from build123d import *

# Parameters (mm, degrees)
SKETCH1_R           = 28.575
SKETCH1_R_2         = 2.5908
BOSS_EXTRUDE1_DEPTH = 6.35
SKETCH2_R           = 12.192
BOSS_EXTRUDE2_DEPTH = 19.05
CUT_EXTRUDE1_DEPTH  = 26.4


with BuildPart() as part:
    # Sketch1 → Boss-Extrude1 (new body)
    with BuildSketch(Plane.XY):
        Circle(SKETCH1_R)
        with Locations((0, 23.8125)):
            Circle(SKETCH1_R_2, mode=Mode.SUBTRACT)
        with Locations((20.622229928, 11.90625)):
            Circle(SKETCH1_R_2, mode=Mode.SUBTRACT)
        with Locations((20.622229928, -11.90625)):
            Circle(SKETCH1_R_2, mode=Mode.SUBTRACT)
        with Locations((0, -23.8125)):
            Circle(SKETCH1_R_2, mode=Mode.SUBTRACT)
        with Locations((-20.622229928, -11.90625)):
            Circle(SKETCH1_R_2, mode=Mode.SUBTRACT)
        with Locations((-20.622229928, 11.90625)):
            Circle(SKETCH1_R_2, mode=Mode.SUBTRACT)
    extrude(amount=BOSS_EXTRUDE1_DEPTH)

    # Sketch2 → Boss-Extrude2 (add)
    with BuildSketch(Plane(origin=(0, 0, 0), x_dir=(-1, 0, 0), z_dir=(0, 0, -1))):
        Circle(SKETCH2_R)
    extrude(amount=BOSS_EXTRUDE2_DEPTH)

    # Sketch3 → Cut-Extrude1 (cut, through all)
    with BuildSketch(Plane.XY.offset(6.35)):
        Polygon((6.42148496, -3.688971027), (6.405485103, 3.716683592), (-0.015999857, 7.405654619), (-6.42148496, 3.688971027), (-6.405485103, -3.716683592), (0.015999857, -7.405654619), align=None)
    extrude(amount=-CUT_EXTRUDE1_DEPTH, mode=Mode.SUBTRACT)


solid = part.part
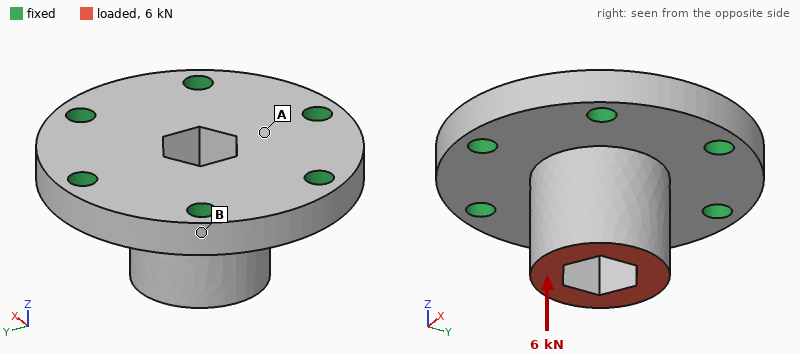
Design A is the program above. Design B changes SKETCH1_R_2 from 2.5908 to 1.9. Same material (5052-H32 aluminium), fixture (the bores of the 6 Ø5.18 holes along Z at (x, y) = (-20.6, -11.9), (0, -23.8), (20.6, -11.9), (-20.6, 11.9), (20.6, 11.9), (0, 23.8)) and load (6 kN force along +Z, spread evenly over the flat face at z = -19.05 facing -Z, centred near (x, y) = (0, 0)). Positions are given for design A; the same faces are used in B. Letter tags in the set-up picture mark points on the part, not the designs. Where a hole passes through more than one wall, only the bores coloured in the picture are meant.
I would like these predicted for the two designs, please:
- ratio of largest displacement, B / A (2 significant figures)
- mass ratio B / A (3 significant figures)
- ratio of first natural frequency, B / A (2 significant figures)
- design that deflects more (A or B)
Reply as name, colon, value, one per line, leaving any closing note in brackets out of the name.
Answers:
ratio of largest displacement, B / A: 1.1
mass ratio B / A: 1.02
ratio of first natural frequency, B / A: 0.96
design that deflects more: B
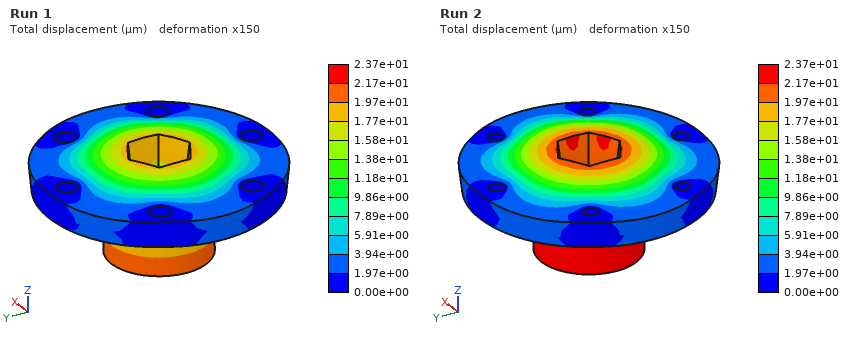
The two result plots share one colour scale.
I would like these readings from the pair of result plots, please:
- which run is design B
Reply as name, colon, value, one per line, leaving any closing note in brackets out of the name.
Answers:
which run is design B: Run 2
